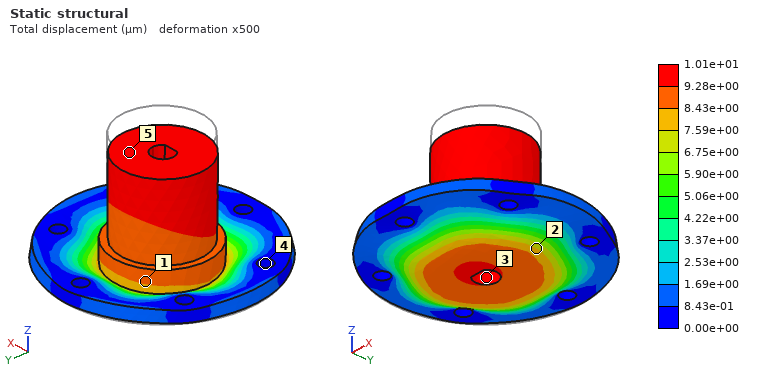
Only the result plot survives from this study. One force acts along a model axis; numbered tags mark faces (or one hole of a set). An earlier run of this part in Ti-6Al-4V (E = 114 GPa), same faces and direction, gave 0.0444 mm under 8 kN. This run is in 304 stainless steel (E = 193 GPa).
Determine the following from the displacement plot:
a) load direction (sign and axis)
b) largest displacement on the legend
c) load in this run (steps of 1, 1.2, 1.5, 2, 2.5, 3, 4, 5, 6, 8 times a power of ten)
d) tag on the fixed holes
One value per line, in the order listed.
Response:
-Z
1.01e+01 µm
3 kN
4
